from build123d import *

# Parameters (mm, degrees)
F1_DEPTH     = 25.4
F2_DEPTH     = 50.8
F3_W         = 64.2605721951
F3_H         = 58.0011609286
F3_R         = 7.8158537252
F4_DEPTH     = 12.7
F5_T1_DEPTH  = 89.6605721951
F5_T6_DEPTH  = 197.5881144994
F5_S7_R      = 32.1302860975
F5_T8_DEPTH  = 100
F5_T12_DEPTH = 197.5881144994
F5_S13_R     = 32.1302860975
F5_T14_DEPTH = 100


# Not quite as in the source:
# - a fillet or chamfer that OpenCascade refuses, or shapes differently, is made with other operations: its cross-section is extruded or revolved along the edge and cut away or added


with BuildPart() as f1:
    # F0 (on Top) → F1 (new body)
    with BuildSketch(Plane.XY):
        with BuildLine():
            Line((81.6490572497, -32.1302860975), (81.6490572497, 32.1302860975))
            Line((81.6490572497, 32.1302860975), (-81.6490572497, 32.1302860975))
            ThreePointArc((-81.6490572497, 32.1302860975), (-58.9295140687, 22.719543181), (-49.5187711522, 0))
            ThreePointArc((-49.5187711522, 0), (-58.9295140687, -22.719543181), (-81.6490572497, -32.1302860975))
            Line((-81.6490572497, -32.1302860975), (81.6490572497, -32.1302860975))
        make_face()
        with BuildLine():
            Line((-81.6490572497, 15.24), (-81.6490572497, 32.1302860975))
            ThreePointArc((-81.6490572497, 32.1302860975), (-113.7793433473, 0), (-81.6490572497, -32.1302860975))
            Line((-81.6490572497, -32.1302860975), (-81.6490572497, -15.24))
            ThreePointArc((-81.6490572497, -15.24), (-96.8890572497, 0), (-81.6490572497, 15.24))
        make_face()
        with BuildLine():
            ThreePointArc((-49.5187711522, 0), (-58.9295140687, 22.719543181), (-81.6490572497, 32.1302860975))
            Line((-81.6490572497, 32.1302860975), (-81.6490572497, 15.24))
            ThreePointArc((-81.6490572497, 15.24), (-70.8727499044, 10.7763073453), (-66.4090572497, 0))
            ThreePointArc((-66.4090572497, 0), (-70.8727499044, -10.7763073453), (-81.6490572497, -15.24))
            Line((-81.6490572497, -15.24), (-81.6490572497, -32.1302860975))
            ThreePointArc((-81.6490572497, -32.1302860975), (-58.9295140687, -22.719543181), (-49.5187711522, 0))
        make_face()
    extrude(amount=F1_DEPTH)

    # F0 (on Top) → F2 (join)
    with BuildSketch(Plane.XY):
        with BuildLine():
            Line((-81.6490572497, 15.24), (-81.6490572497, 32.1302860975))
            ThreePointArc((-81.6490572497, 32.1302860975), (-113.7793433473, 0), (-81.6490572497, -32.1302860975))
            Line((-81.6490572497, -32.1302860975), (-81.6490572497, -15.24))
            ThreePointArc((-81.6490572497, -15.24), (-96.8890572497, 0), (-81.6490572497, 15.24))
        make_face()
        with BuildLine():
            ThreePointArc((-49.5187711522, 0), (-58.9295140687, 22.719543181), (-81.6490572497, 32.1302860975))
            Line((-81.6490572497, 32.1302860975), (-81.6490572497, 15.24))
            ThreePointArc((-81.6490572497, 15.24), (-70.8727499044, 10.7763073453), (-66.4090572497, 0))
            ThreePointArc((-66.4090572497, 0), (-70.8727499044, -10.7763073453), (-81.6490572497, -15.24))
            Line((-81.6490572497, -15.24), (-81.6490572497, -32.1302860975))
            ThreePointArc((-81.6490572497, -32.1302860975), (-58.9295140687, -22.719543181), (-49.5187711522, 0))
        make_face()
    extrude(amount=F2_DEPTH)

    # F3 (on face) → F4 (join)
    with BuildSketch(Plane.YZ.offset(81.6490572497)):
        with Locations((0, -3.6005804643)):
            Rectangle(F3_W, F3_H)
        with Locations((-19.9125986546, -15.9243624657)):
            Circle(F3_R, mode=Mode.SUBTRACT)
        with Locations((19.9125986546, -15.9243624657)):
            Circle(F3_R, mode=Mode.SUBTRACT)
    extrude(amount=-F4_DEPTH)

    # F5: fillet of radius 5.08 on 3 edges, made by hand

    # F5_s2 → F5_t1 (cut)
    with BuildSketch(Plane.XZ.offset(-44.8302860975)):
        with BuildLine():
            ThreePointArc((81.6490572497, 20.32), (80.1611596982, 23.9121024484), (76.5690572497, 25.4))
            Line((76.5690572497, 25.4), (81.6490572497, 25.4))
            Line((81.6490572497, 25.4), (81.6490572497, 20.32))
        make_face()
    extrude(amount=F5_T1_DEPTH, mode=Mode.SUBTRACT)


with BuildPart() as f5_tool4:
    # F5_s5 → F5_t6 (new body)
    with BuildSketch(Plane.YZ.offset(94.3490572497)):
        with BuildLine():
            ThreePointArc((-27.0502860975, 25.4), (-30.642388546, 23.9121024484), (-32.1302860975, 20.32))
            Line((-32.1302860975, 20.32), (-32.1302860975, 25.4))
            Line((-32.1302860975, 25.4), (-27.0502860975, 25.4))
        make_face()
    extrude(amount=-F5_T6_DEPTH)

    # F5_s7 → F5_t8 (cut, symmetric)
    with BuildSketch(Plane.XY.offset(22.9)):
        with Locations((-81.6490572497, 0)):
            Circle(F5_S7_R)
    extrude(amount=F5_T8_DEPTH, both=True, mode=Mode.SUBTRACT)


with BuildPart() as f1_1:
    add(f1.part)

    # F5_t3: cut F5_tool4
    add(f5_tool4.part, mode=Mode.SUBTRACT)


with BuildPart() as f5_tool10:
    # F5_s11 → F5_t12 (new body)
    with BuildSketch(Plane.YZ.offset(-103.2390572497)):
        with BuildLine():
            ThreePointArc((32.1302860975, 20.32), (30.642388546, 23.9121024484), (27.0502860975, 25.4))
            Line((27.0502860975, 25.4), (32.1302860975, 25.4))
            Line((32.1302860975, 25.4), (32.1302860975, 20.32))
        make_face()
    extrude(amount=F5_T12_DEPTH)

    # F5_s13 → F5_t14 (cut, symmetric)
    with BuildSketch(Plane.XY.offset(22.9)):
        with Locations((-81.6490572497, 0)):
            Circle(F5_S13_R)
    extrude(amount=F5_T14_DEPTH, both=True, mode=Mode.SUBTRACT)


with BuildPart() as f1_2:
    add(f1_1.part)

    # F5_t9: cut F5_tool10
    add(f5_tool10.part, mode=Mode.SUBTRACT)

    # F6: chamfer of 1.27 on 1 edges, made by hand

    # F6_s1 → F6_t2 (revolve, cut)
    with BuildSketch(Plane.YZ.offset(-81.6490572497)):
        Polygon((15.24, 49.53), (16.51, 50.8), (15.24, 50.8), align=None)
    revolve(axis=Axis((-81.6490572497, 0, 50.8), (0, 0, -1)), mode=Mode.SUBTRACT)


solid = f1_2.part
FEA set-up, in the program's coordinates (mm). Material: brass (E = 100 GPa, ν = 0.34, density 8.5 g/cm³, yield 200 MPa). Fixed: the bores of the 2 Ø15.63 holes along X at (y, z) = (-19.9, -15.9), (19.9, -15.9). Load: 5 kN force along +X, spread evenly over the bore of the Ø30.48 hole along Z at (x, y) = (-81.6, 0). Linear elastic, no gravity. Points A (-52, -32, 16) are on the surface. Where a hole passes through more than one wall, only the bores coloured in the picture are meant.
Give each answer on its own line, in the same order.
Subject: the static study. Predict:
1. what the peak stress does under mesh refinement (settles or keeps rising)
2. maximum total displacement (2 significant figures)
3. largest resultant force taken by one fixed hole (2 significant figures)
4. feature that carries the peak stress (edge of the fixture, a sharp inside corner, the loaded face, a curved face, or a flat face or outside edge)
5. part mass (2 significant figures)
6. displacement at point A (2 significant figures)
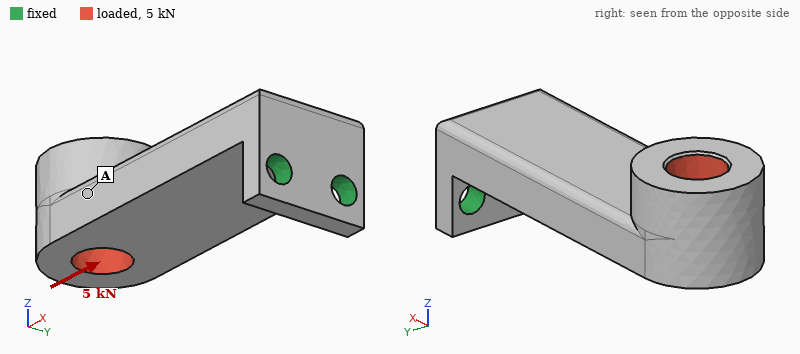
keeps rising
0.53 mm
2.5 kN
edge of the fixture
3.2 kg
0.32 mm
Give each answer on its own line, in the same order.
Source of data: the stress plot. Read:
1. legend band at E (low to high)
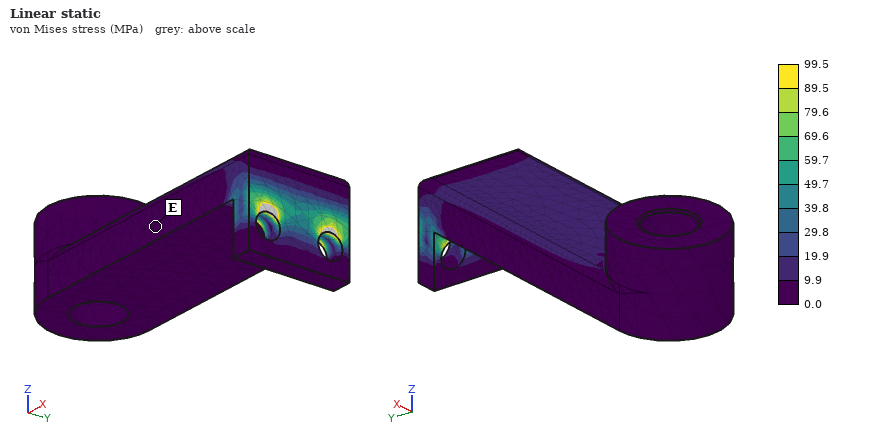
0.0 to 9.9 MPa
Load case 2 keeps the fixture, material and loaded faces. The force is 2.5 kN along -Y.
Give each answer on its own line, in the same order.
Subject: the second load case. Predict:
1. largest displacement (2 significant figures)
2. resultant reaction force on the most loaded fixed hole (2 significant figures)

0.26 mm
8.7 kN
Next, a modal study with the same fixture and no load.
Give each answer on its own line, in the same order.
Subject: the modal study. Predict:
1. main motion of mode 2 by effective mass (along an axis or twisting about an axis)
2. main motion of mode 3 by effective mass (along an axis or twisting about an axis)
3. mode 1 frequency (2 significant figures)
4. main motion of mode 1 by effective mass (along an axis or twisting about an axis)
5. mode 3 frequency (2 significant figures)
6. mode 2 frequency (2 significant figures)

along Y
twisting about X
180 Hz
along Z
1400 Hz
440 Hz
